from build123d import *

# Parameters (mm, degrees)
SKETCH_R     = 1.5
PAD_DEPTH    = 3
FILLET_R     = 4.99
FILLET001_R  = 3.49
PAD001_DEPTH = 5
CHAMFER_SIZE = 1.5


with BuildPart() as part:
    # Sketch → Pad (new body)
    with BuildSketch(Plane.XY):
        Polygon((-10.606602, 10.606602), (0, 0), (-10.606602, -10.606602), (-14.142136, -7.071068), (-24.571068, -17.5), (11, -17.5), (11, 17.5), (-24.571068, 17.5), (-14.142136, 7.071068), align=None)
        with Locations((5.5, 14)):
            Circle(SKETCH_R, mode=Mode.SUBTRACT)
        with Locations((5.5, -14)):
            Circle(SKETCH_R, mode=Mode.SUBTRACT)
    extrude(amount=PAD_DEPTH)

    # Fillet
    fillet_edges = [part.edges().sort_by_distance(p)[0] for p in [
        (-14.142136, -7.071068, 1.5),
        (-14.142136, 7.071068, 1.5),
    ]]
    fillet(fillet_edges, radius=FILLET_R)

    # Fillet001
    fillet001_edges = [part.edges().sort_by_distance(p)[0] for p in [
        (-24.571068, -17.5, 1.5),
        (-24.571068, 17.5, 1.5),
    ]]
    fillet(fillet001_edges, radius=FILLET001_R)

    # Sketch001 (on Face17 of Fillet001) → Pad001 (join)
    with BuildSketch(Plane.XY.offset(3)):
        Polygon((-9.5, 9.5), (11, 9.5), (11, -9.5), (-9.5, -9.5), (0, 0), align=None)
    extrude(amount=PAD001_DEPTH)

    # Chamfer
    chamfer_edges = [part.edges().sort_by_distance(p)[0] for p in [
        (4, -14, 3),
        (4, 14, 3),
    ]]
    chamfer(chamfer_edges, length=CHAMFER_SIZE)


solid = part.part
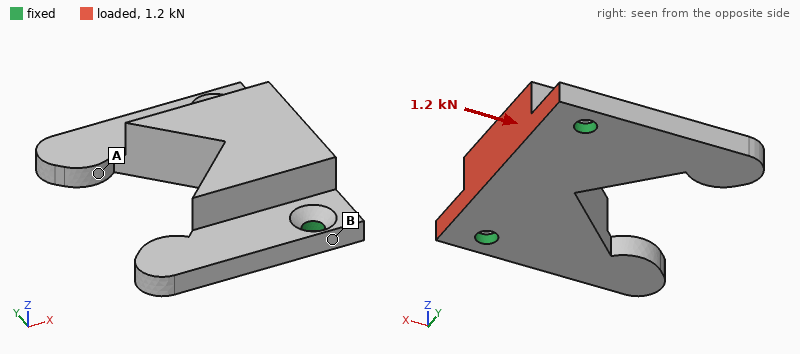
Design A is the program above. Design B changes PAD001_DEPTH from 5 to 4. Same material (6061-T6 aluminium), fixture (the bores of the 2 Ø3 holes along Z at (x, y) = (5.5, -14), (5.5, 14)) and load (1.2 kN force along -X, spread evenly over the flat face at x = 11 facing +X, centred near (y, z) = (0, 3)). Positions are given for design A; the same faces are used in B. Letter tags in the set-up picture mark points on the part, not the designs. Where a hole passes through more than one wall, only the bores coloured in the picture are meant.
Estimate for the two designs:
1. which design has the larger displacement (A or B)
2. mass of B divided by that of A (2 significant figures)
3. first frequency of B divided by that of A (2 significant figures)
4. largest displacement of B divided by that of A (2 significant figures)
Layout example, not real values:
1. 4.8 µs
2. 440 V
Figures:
1. A
2. 0.92
3. 1.0
4. 0.83
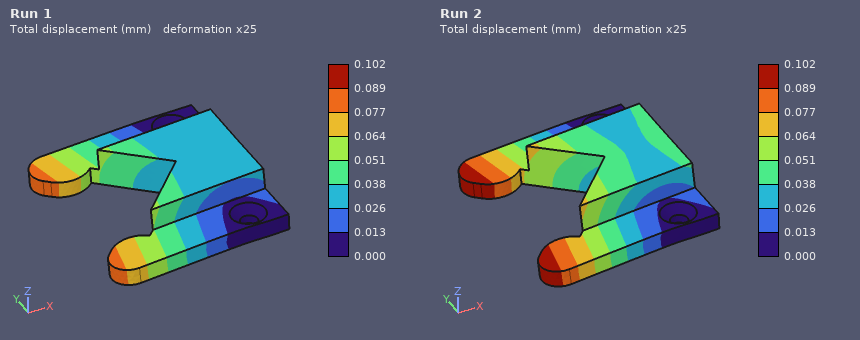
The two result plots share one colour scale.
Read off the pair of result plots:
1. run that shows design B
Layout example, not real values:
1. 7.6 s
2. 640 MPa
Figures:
1. Run 1
